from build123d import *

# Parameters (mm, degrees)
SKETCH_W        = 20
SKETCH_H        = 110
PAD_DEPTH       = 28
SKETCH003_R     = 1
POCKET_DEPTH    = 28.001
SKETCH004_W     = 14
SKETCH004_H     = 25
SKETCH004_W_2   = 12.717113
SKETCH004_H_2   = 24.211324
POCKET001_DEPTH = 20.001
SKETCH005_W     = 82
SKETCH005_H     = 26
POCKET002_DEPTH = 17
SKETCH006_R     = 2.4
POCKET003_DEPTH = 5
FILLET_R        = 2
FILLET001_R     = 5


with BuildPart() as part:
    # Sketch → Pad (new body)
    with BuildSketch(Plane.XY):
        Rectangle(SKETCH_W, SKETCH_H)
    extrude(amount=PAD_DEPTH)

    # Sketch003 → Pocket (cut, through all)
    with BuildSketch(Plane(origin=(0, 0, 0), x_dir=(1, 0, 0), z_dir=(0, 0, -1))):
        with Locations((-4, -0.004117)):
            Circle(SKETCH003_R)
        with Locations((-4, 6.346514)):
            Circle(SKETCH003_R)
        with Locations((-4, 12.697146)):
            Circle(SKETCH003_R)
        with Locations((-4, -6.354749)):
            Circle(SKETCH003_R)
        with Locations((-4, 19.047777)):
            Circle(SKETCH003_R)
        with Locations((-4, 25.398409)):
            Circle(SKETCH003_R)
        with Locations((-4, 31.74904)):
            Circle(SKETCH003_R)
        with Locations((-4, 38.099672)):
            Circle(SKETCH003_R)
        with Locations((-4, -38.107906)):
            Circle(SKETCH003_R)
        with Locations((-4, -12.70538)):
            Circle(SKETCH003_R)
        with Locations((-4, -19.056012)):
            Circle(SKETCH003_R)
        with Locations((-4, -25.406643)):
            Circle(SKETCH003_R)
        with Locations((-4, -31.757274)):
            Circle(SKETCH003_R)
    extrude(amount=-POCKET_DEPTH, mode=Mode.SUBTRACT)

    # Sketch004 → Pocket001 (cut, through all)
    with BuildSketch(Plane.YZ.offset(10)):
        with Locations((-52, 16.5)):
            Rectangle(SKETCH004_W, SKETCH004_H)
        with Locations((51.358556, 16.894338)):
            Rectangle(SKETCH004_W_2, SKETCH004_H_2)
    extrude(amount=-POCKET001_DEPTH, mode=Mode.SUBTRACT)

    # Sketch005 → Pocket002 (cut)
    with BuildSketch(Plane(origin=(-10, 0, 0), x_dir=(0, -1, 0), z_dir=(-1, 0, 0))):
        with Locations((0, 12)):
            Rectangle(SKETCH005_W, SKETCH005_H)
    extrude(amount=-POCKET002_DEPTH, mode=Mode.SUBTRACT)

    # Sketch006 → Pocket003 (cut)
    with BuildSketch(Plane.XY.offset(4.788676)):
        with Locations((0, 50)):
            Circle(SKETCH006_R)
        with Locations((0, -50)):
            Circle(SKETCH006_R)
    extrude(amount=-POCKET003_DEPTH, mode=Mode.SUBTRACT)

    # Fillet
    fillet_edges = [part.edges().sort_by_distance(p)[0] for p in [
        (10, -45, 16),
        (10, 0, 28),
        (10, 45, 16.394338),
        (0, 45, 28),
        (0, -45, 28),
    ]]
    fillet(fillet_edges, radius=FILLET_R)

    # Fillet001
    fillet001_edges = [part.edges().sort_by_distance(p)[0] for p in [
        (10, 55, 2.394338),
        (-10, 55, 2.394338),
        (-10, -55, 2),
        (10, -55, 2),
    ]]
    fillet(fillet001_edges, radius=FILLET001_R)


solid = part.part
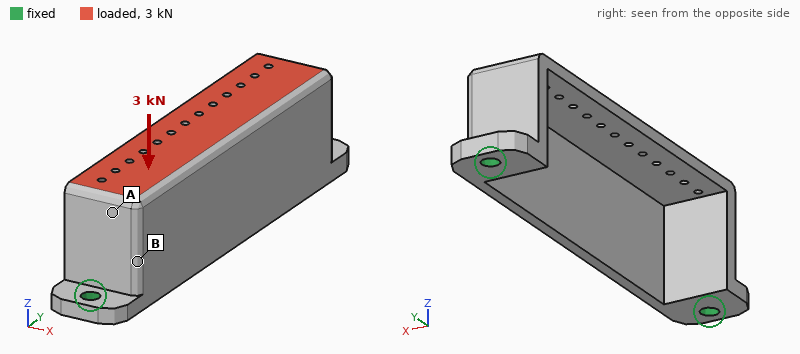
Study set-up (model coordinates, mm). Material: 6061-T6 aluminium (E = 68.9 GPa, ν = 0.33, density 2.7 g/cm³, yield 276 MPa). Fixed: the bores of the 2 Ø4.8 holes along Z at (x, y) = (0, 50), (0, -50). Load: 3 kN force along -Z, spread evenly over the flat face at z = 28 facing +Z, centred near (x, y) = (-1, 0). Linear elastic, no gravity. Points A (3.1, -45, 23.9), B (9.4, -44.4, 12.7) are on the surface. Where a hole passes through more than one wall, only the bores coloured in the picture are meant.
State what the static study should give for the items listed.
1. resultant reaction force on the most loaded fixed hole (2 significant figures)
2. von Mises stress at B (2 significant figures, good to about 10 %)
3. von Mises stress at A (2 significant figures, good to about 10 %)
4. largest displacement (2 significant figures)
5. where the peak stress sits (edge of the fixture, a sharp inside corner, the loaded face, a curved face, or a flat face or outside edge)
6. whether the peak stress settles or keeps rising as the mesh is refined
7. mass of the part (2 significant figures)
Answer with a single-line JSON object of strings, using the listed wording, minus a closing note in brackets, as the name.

{"resultant reaction force on the most loaded fixed hole": "1.7 kN", "von Mises stress at B": "19 MPa", "von Mises stress at A": "34 MPa", "largest displacement": "0.51 mm", "where the peak stress sits": "a sharp inside corner", "whether the peak stress settles or keeps rising as the mesh is refined": "keeps rising", "mass of the part": "45 g"}
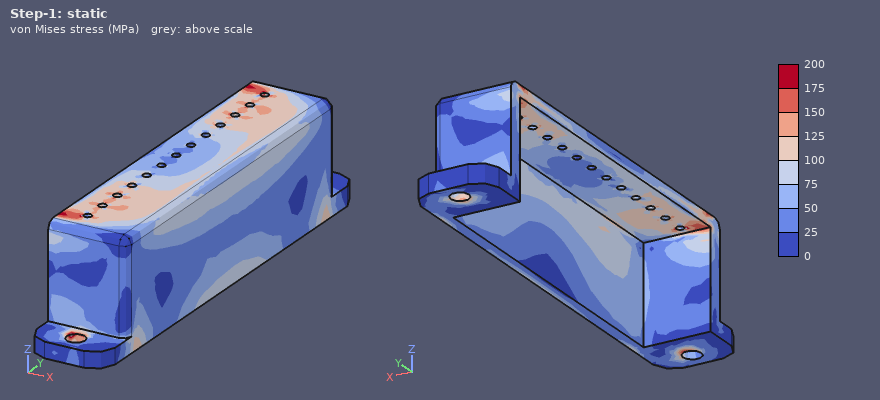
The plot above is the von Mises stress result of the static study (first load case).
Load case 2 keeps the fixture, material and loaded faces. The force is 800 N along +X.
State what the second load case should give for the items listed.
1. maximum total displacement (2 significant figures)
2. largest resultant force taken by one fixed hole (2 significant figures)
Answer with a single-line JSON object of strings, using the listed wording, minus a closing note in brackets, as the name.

{"maximum total displacement": "0.17 mm", "largest resultant force taken by one fixed hole": "420 N"}
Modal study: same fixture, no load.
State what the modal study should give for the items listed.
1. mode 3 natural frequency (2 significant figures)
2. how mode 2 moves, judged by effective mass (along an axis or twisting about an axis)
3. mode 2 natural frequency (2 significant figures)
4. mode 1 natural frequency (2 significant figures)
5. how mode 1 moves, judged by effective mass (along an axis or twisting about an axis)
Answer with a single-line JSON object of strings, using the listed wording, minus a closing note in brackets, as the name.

{"mode 3 natural frequency": "4200 Hz", "how mode 2 moves, judged by effective mass": "twisting about Y", "mode 2 natural frequency": "3300 Hz", "mode 1 natural frequency": "2600 Hz", "how mode 1 moves, judged by effective mass": "along X"}
